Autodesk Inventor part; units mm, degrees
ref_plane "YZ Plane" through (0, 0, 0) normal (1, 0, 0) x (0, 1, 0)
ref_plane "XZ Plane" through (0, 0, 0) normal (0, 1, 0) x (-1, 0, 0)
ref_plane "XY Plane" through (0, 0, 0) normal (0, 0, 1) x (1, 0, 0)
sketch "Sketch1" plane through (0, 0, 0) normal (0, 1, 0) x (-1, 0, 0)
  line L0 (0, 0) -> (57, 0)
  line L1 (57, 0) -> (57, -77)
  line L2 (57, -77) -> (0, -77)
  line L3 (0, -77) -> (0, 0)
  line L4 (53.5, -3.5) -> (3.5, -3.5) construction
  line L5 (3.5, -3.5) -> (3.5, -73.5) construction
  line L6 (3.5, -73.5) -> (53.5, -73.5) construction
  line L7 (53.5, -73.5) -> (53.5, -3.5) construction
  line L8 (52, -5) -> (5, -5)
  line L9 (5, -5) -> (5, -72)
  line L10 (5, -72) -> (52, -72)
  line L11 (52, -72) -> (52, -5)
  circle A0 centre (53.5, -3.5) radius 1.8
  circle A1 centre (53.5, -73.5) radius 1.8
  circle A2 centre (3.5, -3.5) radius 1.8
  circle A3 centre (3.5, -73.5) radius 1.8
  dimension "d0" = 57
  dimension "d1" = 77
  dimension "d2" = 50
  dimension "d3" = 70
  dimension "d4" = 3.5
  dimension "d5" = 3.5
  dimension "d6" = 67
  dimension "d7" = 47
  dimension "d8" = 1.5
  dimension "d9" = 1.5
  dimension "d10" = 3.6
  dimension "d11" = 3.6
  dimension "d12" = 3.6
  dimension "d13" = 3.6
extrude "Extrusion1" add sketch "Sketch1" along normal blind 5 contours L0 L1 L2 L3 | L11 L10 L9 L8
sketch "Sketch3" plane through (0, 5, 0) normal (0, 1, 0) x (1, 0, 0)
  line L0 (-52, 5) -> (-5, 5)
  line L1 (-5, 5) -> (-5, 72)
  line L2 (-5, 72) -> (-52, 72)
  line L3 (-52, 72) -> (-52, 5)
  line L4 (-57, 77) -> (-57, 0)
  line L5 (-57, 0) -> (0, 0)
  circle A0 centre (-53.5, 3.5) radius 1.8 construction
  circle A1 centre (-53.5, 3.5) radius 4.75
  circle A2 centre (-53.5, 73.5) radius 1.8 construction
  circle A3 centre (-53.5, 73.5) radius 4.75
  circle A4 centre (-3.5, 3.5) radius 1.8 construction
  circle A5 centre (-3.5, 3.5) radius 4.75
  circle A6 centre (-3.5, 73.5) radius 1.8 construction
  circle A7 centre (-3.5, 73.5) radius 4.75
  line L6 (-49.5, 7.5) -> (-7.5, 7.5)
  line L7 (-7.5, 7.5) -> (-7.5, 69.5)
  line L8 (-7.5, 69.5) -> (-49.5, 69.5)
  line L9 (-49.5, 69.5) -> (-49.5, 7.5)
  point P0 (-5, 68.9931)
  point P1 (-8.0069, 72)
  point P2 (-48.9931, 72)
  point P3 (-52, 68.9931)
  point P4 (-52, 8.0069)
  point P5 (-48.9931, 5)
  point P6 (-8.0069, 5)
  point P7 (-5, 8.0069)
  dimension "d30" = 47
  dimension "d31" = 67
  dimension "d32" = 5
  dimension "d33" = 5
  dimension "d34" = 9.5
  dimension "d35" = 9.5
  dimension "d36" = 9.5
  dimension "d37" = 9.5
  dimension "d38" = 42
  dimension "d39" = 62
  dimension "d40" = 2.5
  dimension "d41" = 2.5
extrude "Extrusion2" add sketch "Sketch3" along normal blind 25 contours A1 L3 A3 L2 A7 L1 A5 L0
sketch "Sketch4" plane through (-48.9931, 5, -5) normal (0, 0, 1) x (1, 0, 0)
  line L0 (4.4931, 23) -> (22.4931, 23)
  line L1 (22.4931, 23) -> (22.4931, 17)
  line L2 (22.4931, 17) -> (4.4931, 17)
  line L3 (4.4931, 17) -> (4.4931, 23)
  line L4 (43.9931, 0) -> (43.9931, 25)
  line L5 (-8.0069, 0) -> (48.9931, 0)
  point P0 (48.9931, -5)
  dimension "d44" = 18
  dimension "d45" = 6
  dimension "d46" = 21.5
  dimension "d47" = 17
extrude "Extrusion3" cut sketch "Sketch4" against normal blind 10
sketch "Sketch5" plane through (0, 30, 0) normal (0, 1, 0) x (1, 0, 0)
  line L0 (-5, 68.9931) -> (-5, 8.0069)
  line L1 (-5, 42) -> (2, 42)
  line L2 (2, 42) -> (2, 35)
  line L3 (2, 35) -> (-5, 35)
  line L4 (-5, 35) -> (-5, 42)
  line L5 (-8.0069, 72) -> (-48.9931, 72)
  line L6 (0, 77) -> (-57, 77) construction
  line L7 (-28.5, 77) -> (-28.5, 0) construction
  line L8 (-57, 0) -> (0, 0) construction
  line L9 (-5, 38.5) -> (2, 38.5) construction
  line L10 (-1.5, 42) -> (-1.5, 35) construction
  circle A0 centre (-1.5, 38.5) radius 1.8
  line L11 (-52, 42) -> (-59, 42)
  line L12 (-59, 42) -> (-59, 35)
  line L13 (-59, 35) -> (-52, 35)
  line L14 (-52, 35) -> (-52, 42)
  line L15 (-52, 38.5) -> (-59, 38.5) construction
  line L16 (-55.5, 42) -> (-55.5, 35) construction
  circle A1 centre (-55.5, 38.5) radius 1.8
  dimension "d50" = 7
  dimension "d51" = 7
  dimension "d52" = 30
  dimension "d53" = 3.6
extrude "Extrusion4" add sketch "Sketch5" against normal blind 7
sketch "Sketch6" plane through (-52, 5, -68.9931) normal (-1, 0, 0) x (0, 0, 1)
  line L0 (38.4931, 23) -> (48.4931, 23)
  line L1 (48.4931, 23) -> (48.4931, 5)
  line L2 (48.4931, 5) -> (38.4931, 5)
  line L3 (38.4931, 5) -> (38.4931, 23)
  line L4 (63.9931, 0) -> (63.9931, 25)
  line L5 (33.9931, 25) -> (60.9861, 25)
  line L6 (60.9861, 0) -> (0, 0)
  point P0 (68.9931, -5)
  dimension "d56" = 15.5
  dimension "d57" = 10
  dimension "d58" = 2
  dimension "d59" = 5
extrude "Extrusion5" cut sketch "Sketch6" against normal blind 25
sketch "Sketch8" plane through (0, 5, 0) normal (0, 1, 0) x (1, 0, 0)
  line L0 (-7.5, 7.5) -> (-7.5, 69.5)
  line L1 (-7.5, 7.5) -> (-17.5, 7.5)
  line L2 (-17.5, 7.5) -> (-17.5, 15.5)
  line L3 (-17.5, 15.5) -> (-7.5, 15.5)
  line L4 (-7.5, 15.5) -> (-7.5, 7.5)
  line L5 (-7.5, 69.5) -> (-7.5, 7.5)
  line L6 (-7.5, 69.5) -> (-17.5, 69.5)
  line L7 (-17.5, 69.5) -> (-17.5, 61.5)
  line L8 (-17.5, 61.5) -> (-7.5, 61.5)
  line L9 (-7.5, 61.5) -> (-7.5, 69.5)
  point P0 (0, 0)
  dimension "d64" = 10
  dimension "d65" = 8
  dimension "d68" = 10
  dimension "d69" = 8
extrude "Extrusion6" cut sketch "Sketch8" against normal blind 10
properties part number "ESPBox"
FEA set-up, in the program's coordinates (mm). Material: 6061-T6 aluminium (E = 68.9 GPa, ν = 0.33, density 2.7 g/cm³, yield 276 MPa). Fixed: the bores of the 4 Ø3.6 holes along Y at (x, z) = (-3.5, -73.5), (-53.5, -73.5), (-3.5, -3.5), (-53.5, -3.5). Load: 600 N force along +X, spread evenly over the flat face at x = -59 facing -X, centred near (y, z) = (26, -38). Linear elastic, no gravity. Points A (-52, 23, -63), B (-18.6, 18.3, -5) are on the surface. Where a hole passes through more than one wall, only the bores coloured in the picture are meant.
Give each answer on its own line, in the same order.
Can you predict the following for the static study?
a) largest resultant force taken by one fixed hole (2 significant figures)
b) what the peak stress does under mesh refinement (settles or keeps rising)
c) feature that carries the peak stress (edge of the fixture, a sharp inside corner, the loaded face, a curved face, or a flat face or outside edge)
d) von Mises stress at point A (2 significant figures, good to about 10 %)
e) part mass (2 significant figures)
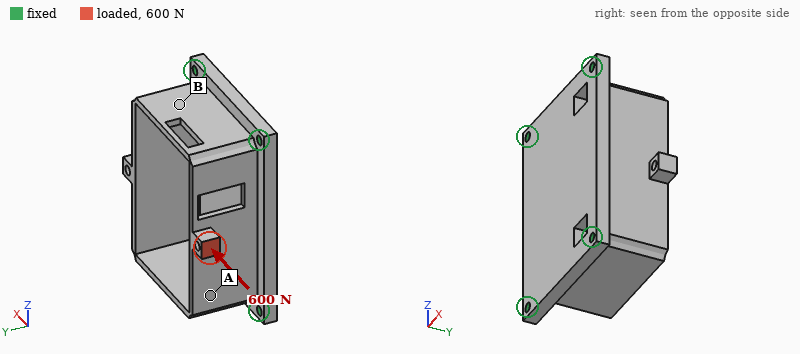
270 N
keeps rising
a sharp inside corner
110 MPa
91 g
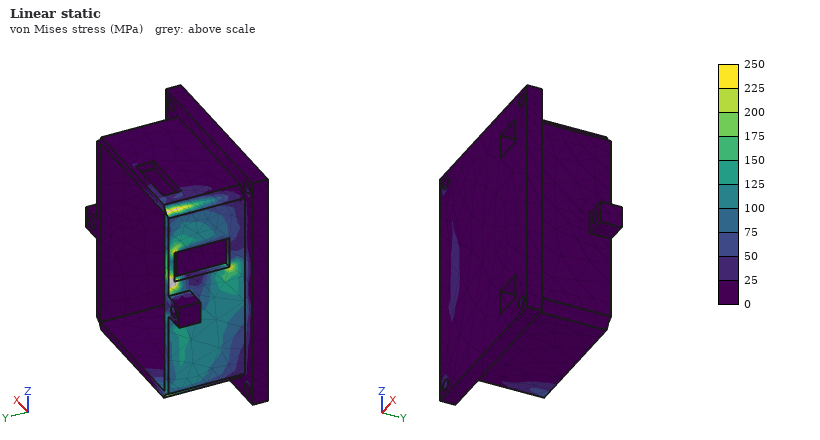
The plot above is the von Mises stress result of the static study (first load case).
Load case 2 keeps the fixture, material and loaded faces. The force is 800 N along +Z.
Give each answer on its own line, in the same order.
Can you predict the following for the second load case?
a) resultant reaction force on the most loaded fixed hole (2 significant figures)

430 N
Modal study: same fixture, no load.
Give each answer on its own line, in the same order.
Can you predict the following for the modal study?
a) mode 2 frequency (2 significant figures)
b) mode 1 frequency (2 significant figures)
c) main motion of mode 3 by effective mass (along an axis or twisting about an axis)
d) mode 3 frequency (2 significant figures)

3800 Hz
3600 Hz
along Y
5900 Hz
